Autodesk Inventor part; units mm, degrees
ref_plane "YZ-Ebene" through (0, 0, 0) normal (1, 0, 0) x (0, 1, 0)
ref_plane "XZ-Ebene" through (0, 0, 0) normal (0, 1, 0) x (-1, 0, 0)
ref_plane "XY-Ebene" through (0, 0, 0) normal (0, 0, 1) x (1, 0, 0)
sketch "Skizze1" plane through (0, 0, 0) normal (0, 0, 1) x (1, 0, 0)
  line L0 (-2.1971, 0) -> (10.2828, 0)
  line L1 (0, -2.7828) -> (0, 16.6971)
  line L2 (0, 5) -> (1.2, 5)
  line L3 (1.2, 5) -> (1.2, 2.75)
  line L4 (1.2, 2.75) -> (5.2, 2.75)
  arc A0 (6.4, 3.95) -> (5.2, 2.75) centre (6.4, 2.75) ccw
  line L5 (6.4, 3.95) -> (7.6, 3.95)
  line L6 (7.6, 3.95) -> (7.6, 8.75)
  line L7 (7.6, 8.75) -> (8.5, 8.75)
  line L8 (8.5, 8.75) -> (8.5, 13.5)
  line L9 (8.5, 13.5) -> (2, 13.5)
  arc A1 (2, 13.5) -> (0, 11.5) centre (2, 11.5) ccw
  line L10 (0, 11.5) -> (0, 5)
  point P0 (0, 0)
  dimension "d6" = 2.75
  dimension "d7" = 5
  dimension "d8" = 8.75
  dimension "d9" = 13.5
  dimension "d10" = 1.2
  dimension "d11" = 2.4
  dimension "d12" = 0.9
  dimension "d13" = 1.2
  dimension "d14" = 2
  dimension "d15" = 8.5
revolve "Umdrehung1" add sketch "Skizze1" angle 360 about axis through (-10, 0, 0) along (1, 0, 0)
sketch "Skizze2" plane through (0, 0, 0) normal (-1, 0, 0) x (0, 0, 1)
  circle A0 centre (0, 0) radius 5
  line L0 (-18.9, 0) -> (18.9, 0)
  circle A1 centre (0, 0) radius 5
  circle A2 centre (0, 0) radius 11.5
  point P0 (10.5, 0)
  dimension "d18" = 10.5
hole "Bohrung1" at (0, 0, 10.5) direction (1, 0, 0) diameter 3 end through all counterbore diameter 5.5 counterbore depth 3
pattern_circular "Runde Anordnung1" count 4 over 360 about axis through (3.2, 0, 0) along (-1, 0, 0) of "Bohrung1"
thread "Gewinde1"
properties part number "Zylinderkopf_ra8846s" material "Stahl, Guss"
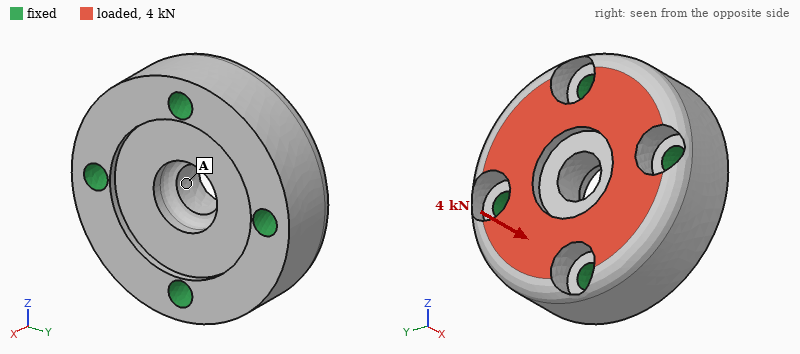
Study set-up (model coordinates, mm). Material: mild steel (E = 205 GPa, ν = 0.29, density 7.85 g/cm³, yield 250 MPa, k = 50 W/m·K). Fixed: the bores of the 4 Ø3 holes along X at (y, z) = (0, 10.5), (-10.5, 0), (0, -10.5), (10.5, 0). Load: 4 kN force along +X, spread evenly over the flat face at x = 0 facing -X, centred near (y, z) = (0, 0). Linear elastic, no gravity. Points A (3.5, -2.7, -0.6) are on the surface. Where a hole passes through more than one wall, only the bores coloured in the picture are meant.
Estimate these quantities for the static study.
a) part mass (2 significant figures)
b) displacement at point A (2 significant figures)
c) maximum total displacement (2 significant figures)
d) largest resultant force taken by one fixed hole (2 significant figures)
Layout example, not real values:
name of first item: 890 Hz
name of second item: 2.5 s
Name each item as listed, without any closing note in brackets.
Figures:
part mass: 30 g
displacement at point A: 1.1 µm
maximum total displacement: 1.2 µm
largest resultant force taken by one fixed hole: 1.0 kN
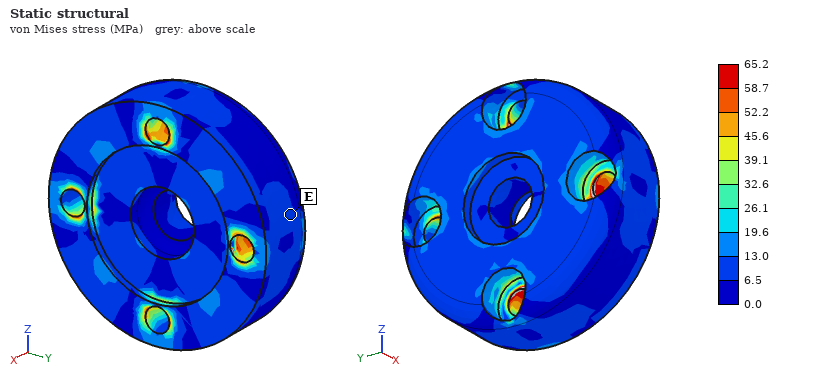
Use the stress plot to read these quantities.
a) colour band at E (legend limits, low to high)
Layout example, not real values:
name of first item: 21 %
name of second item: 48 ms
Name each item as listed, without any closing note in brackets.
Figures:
colour band at E: 6.5 to 13.0 MPa
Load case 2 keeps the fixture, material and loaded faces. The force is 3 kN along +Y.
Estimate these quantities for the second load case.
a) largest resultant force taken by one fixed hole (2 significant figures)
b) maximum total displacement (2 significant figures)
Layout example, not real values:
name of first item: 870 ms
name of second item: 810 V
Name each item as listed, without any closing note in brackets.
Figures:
largest resultant force taken by one fixed hole: 1.0 kN
maximum total displacement: 1.5 µm
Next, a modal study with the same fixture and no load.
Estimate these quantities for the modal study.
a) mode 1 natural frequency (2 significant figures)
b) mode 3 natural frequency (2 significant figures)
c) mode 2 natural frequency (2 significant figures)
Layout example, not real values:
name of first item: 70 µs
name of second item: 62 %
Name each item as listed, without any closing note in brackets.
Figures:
mode 1 natural frequency: 63 kHz
mode 3 natural frequency: 65 kHz
mode 2 natural frequency: 65 kHz
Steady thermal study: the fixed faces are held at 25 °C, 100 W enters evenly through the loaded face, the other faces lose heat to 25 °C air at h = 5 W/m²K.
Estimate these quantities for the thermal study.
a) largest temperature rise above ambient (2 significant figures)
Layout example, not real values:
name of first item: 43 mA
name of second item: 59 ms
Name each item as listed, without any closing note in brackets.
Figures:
largest temperature rise above ambient: 50 K
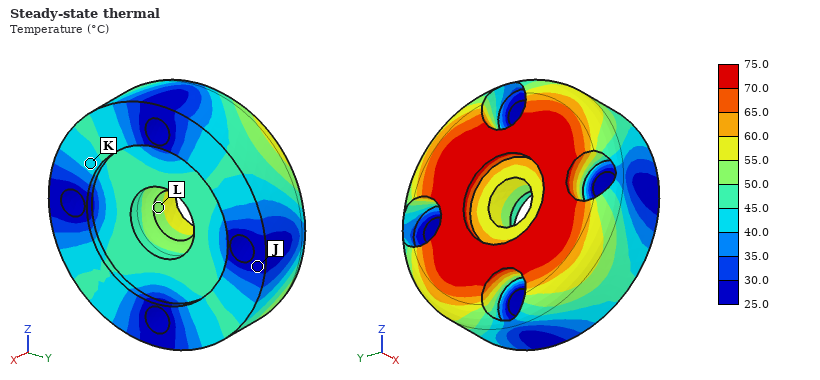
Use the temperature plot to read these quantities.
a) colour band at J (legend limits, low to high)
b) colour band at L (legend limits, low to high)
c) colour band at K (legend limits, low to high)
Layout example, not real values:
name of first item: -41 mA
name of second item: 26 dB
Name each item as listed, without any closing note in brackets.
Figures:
colour band at J: 25.0 to 30.0 °C
colour band at L: 50.0 to 55.0 °C
colour band at K: 40.0 to 45.0 °C
